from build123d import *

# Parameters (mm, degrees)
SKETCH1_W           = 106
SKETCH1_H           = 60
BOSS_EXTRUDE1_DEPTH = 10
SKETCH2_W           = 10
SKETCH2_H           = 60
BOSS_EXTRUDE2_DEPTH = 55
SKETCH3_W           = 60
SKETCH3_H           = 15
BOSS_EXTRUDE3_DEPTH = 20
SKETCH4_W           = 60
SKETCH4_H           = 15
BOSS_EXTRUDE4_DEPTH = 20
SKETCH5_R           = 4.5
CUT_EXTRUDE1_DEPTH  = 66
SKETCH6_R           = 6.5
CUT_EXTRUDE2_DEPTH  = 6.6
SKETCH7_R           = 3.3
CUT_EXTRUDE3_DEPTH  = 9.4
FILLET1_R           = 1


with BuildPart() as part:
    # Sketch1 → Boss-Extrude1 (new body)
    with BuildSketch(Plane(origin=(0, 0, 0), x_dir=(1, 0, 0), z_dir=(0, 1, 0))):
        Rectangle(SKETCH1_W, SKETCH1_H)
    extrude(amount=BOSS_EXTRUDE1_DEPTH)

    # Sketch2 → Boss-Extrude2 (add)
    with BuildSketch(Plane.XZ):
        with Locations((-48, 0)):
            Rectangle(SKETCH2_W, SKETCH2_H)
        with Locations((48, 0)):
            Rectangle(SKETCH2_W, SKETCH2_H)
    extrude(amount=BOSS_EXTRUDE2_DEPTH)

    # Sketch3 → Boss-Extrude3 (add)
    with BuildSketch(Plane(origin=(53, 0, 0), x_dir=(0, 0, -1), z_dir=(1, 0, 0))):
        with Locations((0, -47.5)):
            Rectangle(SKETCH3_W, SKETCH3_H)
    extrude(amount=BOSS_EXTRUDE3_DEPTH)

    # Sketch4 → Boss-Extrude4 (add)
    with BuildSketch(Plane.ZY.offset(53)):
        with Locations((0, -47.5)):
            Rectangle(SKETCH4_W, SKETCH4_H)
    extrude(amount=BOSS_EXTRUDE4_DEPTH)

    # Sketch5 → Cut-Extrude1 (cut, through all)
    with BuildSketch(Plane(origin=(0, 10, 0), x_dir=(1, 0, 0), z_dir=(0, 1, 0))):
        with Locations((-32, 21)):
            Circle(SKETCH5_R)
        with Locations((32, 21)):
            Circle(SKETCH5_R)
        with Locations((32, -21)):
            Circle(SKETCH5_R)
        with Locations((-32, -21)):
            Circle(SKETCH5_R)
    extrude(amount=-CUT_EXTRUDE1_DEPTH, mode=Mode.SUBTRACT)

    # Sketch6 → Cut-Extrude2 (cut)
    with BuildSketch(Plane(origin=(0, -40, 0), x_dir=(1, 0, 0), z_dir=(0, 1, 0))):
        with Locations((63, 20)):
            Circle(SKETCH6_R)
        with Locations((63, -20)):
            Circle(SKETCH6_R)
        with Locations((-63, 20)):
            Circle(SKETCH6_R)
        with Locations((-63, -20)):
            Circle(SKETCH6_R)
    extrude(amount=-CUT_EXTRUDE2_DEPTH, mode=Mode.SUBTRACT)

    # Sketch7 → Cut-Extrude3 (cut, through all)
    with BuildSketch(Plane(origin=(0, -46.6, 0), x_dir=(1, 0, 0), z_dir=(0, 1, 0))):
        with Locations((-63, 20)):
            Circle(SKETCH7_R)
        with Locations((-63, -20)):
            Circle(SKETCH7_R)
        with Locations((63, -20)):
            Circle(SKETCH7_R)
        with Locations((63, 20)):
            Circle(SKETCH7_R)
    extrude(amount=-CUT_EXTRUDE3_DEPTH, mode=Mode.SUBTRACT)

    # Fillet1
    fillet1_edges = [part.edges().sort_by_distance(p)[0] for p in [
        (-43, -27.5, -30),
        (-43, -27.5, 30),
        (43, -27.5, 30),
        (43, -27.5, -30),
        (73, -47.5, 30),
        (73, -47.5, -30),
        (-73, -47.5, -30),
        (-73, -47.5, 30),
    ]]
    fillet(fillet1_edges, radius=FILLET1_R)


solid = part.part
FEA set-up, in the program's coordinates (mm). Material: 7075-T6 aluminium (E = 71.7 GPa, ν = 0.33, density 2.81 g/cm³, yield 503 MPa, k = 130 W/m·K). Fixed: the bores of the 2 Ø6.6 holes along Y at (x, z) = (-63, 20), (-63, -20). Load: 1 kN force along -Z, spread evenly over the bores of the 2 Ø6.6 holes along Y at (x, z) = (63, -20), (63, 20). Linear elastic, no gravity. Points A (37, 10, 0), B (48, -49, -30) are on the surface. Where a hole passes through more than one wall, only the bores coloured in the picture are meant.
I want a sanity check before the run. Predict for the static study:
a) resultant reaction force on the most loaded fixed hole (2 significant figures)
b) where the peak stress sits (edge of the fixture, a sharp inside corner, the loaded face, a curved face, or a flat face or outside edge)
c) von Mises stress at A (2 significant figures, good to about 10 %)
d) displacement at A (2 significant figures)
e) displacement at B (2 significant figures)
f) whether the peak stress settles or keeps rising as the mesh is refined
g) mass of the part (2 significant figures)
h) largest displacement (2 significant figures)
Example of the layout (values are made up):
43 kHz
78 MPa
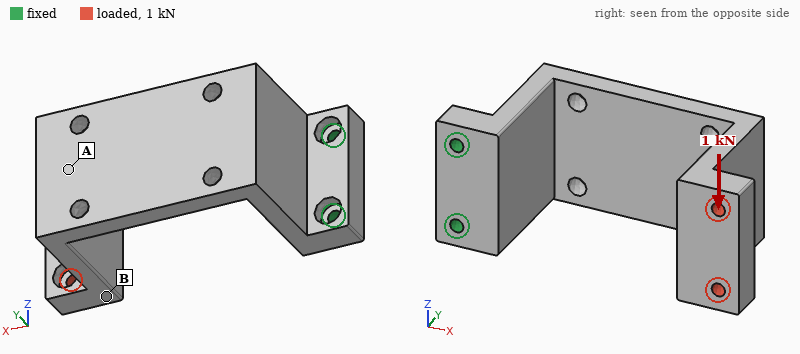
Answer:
2.8 kN
edge of the fixture
32 MPa
0.68 mm
1.6 mm
keeps rising
440 g
1.9 mm
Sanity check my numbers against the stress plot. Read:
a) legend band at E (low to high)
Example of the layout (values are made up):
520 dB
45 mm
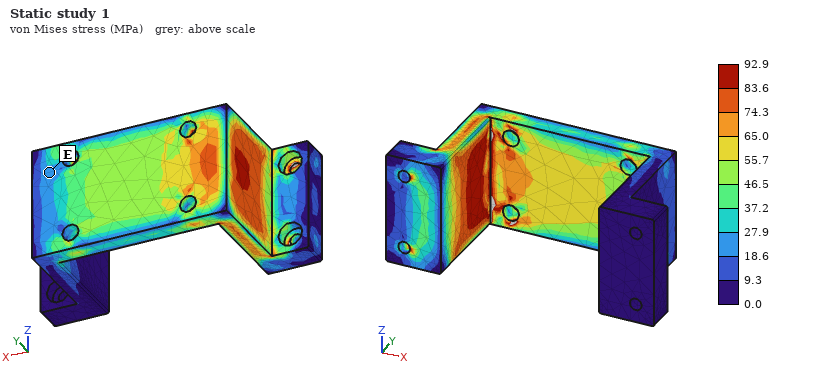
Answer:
18.6 to 27.9 MPa
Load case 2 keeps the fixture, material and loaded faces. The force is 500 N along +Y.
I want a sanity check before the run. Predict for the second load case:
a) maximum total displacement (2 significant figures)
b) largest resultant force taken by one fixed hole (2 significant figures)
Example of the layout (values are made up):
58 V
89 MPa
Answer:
2.0 mm
370 N
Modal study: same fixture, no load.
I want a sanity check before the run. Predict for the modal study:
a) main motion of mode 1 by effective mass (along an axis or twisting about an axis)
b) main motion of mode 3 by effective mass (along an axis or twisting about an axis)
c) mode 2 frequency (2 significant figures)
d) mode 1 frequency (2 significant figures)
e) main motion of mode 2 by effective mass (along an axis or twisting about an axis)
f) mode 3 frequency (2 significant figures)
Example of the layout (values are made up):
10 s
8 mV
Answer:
along Y
along X
360 Hz
210 Hz
along Z
620 Hz
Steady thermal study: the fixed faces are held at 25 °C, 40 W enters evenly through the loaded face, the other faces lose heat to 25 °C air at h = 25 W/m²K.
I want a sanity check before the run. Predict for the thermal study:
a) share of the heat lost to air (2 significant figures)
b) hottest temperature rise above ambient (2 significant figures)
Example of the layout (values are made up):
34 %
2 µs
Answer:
63 %
62 K
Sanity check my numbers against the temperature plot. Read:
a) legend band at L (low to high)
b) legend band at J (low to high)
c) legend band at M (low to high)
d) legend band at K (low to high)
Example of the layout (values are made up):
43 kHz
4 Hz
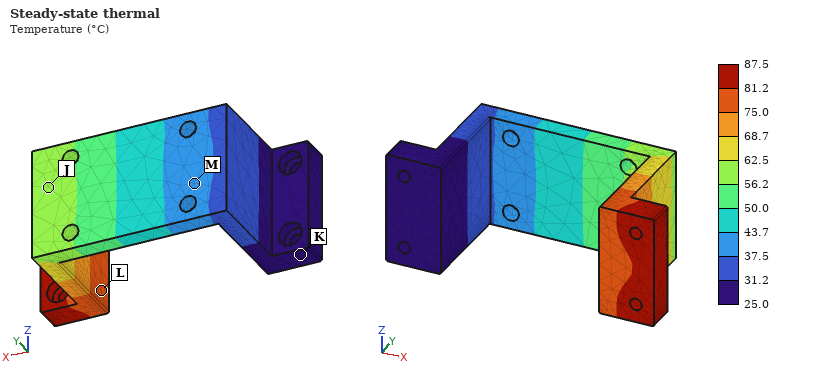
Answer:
75.0 to 81.2 °C
56.2 to 62.5 °C
37.5 to 43.7 °C
25.0 to 31.2 °C
